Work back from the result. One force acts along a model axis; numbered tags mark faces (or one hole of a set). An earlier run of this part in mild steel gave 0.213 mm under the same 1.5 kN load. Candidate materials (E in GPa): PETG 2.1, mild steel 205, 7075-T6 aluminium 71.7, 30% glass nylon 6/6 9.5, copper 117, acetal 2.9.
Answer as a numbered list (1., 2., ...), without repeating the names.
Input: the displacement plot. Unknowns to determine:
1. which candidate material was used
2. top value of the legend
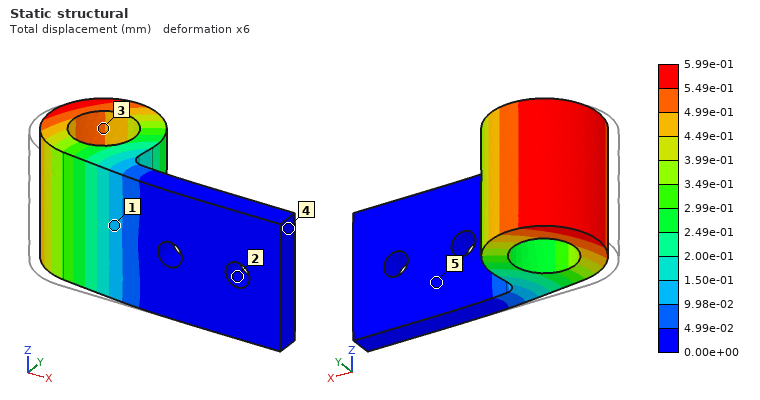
1. 7075-T6 aluminium
2. 5.99e-01 mm
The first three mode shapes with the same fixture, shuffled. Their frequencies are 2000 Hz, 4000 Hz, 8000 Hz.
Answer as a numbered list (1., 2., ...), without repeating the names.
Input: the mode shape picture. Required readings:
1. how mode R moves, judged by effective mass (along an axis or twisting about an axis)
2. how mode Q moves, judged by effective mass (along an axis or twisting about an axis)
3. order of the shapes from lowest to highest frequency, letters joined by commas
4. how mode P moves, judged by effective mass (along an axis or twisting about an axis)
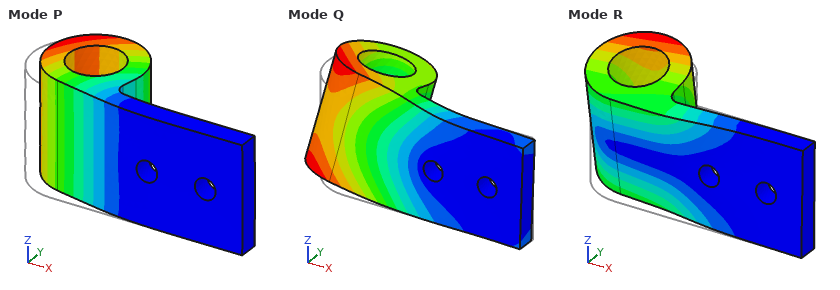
1. along Z
2. along Z
3. P, R, Q
4. along Y
